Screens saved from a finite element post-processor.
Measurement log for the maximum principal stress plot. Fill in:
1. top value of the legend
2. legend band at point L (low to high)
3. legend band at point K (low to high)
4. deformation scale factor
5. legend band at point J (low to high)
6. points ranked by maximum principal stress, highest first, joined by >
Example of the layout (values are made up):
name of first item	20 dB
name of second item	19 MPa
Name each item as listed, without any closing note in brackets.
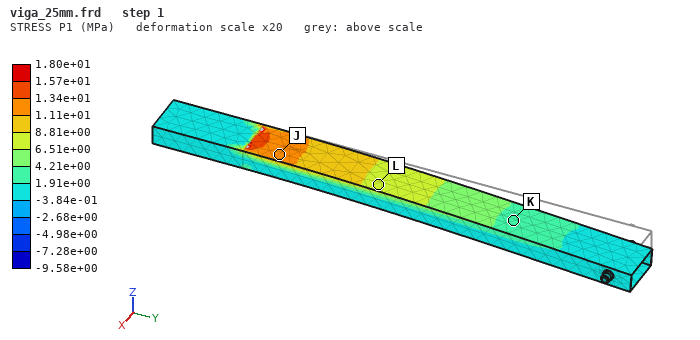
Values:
top value of the legend	1.80e+01 MPa
legend band at point L	6.51e+00 to 8.81e+00 MPa
legend band at point K	1.91e+00 to 4.21e+00 MPa
deformation scale factor	20
legend band at point J	1.11e+01 to 1.34e+01 MPa
points ranked by maximum principal stress, highest first, joined by >	J > L > K
